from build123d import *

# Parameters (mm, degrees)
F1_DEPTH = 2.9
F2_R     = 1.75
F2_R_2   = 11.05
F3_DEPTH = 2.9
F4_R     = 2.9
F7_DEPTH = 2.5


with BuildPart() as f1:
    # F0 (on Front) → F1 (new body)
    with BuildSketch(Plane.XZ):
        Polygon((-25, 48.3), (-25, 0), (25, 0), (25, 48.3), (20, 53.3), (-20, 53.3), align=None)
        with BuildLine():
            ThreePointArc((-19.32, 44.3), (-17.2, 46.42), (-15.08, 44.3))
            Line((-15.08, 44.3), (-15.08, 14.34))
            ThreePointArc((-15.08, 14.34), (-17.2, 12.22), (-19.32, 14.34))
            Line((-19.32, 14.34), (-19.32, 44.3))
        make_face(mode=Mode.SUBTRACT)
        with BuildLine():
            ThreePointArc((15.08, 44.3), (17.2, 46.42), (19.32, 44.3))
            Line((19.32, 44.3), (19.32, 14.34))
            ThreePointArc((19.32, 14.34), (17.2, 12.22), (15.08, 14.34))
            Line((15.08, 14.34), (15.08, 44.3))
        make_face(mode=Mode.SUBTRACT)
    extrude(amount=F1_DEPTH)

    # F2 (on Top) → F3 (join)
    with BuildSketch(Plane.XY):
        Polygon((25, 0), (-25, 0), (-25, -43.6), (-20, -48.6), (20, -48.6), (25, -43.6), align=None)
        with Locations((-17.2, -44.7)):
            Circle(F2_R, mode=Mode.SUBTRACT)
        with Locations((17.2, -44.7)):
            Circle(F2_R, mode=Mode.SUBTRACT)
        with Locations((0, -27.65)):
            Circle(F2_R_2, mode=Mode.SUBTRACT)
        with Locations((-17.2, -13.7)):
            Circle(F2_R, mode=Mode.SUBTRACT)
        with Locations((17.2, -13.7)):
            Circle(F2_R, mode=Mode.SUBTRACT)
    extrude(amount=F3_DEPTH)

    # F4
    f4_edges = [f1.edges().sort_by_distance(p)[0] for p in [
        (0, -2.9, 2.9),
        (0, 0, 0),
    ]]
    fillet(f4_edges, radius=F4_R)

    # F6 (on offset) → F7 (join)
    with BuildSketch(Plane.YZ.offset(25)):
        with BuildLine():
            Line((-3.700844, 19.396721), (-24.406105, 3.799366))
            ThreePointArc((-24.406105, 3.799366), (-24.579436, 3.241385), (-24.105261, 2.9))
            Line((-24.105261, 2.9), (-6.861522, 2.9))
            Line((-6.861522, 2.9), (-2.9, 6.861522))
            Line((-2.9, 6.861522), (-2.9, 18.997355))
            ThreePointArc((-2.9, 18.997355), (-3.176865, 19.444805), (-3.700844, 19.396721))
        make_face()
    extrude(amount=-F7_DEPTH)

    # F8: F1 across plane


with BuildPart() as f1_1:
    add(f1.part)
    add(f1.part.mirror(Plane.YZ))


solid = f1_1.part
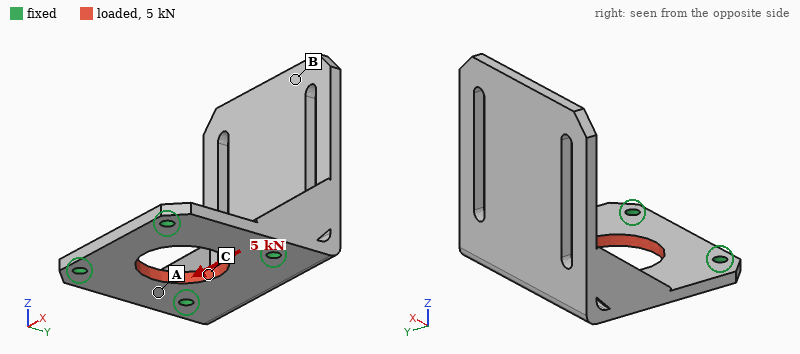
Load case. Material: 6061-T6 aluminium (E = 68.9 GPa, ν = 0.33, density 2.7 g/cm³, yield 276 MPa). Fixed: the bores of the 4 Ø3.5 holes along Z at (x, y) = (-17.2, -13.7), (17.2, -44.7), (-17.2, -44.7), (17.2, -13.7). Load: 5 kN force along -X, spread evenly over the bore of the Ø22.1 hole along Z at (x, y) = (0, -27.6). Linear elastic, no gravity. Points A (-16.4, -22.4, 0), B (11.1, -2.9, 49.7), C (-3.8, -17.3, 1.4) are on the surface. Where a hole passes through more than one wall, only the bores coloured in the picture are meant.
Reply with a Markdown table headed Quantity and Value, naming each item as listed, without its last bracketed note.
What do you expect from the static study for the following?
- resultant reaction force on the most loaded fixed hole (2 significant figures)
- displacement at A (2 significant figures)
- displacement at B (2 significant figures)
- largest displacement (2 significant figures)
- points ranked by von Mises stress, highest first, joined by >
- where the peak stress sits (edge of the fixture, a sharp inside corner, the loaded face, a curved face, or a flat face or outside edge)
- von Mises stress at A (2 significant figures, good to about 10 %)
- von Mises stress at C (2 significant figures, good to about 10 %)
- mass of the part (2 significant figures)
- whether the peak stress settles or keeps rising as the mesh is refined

| Quantity | Value |
|---|---|
| resultant reaction force on the most loaded fixed hole | 1.4 kN |
| displacement at A | 7.8 µm |
| displacement at B | 3.4 µm |
| largest displacement | 12 µm |
| points ranked by von Mises stress, highest first, joined by > | C > A > B |
| where the peak stress sits | edge of the fixture |
| von Mises stress at A | 27 MPa |
| von Mises stress at C | 42 MPa |
| mass of the part | 35 g |
| whether the peak stress settles or keeps rising as the mesh is refined | keeps rising |
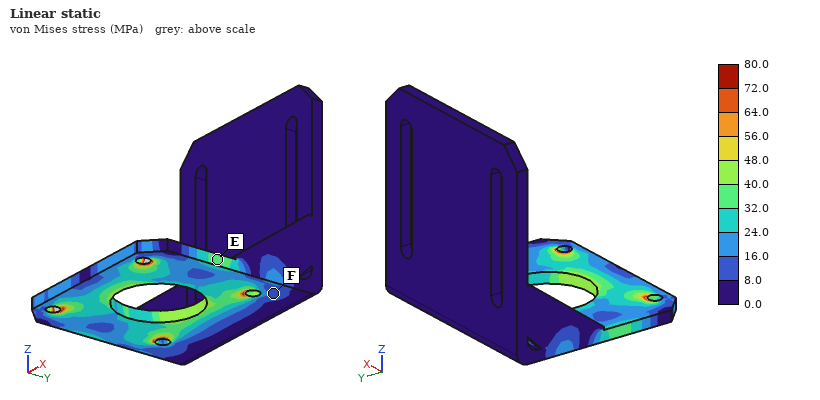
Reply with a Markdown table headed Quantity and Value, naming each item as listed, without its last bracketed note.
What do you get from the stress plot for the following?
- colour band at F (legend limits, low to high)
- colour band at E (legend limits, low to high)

| Quantity | Value |
|---|---|
| colour band at F | 8.0 to 16.0 MPa |
| colour band at E | 32.0 to 40.0 MPa |
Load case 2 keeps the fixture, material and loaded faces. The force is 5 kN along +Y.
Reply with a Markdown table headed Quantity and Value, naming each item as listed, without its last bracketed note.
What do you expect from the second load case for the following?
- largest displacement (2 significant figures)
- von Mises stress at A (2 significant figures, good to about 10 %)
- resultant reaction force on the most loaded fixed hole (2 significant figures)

| Quantity | Value |
|---|---|
| largest displacement | 18 µm |
| von Mises stress at A | 32 MPa |
| resultant reaction force on the most loaded fixed hole | 1.4 kN |
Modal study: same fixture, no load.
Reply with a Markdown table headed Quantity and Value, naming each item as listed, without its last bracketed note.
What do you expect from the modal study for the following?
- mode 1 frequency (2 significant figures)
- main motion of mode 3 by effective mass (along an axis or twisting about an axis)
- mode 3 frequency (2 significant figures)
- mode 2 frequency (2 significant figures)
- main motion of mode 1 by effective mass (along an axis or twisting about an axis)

| Quantity | Value |
|---|---|
| mode 1 frequency | 1000 Hz |
| main motion of mode 3 by effective mass | along X |
| mode 3 frequency | 3600 Hz |
| mode 2 frequency | 2400 Hz |
| main motion of mode 1 by effective mass | along Y |
